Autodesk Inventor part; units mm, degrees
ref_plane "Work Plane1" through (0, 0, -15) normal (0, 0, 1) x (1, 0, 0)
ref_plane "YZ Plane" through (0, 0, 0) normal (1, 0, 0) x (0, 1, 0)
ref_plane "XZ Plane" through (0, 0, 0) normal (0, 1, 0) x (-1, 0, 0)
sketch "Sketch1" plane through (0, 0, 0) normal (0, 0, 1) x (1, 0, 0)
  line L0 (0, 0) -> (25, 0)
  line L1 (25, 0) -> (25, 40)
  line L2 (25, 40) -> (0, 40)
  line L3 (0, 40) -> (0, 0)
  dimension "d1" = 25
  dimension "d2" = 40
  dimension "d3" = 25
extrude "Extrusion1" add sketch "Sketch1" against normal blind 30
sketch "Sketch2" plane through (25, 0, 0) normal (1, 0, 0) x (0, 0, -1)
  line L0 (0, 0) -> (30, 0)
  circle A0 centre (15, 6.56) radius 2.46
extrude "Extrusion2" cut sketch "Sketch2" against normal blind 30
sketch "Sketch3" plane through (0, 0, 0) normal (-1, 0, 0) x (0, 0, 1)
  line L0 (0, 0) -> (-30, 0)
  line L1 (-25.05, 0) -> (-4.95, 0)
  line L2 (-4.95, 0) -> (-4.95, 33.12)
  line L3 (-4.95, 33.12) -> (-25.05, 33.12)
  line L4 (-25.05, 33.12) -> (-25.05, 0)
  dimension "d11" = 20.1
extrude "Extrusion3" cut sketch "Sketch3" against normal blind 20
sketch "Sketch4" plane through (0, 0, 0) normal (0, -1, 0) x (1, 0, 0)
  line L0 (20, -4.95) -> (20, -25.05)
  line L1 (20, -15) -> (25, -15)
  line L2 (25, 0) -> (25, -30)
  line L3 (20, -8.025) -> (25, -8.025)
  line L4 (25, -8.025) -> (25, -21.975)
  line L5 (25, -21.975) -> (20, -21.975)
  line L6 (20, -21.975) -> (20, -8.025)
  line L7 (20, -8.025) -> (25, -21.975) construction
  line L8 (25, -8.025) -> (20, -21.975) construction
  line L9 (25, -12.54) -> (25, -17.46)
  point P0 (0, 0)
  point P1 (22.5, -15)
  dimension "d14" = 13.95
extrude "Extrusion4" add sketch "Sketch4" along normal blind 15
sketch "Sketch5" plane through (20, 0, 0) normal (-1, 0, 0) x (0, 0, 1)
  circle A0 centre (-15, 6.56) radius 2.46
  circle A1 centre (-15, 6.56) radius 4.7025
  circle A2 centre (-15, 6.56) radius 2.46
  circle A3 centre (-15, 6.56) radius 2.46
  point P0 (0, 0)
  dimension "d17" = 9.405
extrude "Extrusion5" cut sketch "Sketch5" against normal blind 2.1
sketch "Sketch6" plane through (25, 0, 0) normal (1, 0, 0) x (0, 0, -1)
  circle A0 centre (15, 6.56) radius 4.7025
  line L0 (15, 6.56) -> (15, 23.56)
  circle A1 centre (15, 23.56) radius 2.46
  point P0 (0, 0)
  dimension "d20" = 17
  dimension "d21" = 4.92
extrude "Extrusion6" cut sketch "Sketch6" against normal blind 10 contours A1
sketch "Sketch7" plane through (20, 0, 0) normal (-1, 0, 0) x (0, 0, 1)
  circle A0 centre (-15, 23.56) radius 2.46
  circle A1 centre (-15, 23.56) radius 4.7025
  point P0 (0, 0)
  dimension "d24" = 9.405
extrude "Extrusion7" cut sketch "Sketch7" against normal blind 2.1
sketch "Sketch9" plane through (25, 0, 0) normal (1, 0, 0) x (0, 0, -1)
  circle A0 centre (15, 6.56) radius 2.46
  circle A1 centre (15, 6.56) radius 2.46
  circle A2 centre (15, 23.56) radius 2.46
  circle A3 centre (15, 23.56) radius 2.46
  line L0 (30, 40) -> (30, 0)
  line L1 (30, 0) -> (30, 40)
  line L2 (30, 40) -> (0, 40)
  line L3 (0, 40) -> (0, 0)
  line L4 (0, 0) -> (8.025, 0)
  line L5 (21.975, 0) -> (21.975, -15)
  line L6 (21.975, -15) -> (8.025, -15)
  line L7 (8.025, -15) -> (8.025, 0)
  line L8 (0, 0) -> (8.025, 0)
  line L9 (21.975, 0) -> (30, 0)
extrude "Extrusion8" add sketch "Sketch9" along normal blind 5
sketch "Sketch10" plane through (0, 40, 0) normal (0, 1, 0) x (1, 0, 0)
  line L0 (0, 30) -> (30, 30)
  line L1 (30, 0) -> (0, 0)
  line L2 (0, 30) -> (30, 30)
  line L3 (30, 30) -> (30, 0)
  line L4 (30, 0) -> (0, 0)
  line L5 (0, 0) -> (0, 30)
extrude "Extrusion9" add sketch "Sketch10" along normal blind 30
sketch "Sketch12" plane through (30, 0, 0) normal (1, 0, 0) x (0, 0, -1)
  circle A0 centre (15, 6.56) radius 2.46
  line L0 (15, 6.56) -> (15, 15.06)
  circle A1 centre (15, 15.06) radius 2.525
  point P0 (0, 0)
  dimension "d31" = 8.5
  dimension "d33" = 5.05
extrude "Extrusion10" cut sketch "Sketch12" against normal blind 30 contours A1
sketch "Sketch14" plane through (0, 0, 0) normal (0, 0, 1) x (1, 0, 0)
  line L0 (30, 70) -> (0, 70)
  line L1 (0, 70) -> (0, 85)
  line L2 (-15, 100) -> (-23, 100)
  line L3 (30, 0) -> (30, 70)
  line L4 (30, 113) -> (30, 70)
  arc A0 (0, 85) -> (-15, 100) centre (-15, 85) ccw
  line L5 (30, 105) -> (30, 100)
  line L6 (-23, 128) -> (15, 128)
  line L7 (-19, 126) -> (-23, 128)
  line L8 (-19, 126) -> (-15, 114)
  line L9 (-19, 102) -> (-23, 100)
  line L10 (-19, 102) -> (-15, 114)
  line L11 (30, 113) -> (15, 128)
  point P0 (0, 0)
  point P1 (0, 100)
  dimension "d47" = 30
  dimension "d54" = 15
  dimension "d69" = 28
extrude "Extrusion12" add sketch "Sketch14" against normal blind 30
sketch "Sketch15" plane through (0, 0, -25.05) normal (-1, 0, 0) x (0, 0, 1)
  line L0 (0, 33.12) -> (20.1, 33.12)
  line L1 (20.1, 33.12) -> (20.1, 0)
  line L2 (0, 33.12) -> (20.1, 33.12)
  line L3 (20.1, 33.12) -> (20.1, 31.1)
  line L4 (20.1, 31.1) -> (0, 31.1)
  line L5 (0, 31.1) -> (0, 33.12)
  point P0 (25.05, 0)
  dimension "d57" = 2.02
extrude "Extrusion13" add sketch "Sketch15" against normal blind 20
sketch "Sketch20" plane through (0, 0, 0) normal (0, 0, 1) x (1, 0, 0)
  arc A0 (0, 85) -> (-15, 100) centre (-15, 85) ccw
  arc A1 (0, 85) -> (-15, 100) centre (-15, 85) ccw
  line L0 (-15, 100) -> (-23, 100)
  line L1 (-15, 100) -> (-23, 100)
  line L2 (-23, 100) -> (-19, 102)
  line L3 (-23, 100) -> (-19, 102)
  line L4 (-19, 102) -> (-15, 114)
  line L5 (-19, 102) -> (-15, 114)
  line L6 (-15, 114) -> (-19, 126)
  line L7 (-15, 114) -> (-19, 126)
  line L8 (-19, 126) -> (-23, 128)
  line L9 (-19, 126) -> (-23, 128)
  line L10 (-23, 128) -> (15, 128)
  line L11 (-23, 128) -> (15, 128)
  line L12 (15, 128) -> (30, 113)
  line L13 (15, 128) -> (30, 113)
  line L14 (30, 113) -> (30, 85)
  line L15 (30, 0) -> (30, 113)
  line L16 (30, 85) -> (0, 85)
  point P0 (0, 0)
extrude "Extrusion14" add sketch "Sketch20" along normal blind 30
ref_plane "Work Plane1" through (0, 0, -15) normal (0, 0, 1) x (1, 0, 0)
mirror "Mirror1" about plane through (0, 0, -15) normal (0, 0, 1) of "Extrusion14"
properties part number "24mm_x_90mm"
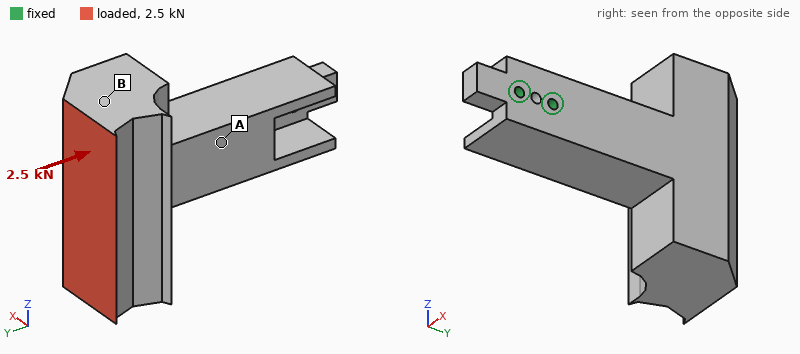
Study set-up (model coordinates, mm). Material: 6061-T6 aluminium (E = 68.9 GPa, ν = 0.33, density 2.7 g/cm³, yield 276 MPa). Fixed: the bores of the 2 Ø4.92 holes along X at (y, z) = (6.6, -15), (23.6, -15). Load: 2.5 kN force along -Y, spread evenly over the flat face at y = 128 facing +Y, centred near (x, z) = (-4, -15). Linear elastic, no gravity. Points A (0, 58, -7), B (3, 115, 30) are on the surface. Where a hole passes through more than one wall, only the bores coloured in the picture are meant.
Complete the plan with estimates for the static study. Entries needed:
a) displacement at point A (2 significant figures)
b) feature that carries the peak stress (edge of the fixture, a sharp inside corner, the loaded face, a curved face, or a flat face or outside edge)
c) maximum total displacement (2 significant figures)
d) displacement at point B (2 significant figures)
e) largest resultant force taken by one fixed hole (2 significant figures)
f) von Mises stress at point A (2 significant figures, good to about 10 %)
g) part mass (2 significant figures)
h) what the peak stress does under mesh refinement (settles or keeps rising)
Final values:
0.077 mm
edge of the fixture
0.24 mm
0.19 mm
3.4 kN
13 MPa
590 g
keeps rising
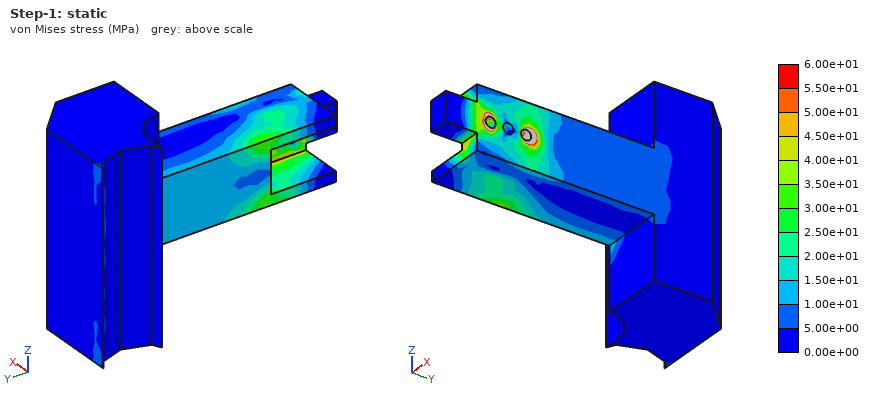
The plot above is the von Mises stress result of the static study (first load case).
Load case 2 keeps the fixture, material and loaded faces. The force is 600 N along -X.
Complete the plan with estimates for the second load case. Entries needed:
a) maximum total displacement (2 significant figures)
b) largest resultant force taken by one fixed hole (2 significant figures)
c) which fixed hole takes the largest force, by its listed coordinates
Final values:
0.21 mm
3.1 kN
(23.6, -15)
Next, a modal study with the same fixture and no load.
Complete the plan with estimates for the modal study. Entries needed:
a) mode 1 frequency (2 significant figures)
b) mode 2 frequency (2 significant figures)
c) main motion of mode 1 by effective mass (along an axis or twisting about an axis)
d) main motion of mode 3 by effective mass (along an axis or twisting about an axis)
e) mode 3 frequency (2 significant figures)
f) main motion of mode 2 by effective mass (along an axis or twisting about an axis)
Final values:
520 Hz
590 Hz
along X
twisting about Y
1000 Hz
along Z
